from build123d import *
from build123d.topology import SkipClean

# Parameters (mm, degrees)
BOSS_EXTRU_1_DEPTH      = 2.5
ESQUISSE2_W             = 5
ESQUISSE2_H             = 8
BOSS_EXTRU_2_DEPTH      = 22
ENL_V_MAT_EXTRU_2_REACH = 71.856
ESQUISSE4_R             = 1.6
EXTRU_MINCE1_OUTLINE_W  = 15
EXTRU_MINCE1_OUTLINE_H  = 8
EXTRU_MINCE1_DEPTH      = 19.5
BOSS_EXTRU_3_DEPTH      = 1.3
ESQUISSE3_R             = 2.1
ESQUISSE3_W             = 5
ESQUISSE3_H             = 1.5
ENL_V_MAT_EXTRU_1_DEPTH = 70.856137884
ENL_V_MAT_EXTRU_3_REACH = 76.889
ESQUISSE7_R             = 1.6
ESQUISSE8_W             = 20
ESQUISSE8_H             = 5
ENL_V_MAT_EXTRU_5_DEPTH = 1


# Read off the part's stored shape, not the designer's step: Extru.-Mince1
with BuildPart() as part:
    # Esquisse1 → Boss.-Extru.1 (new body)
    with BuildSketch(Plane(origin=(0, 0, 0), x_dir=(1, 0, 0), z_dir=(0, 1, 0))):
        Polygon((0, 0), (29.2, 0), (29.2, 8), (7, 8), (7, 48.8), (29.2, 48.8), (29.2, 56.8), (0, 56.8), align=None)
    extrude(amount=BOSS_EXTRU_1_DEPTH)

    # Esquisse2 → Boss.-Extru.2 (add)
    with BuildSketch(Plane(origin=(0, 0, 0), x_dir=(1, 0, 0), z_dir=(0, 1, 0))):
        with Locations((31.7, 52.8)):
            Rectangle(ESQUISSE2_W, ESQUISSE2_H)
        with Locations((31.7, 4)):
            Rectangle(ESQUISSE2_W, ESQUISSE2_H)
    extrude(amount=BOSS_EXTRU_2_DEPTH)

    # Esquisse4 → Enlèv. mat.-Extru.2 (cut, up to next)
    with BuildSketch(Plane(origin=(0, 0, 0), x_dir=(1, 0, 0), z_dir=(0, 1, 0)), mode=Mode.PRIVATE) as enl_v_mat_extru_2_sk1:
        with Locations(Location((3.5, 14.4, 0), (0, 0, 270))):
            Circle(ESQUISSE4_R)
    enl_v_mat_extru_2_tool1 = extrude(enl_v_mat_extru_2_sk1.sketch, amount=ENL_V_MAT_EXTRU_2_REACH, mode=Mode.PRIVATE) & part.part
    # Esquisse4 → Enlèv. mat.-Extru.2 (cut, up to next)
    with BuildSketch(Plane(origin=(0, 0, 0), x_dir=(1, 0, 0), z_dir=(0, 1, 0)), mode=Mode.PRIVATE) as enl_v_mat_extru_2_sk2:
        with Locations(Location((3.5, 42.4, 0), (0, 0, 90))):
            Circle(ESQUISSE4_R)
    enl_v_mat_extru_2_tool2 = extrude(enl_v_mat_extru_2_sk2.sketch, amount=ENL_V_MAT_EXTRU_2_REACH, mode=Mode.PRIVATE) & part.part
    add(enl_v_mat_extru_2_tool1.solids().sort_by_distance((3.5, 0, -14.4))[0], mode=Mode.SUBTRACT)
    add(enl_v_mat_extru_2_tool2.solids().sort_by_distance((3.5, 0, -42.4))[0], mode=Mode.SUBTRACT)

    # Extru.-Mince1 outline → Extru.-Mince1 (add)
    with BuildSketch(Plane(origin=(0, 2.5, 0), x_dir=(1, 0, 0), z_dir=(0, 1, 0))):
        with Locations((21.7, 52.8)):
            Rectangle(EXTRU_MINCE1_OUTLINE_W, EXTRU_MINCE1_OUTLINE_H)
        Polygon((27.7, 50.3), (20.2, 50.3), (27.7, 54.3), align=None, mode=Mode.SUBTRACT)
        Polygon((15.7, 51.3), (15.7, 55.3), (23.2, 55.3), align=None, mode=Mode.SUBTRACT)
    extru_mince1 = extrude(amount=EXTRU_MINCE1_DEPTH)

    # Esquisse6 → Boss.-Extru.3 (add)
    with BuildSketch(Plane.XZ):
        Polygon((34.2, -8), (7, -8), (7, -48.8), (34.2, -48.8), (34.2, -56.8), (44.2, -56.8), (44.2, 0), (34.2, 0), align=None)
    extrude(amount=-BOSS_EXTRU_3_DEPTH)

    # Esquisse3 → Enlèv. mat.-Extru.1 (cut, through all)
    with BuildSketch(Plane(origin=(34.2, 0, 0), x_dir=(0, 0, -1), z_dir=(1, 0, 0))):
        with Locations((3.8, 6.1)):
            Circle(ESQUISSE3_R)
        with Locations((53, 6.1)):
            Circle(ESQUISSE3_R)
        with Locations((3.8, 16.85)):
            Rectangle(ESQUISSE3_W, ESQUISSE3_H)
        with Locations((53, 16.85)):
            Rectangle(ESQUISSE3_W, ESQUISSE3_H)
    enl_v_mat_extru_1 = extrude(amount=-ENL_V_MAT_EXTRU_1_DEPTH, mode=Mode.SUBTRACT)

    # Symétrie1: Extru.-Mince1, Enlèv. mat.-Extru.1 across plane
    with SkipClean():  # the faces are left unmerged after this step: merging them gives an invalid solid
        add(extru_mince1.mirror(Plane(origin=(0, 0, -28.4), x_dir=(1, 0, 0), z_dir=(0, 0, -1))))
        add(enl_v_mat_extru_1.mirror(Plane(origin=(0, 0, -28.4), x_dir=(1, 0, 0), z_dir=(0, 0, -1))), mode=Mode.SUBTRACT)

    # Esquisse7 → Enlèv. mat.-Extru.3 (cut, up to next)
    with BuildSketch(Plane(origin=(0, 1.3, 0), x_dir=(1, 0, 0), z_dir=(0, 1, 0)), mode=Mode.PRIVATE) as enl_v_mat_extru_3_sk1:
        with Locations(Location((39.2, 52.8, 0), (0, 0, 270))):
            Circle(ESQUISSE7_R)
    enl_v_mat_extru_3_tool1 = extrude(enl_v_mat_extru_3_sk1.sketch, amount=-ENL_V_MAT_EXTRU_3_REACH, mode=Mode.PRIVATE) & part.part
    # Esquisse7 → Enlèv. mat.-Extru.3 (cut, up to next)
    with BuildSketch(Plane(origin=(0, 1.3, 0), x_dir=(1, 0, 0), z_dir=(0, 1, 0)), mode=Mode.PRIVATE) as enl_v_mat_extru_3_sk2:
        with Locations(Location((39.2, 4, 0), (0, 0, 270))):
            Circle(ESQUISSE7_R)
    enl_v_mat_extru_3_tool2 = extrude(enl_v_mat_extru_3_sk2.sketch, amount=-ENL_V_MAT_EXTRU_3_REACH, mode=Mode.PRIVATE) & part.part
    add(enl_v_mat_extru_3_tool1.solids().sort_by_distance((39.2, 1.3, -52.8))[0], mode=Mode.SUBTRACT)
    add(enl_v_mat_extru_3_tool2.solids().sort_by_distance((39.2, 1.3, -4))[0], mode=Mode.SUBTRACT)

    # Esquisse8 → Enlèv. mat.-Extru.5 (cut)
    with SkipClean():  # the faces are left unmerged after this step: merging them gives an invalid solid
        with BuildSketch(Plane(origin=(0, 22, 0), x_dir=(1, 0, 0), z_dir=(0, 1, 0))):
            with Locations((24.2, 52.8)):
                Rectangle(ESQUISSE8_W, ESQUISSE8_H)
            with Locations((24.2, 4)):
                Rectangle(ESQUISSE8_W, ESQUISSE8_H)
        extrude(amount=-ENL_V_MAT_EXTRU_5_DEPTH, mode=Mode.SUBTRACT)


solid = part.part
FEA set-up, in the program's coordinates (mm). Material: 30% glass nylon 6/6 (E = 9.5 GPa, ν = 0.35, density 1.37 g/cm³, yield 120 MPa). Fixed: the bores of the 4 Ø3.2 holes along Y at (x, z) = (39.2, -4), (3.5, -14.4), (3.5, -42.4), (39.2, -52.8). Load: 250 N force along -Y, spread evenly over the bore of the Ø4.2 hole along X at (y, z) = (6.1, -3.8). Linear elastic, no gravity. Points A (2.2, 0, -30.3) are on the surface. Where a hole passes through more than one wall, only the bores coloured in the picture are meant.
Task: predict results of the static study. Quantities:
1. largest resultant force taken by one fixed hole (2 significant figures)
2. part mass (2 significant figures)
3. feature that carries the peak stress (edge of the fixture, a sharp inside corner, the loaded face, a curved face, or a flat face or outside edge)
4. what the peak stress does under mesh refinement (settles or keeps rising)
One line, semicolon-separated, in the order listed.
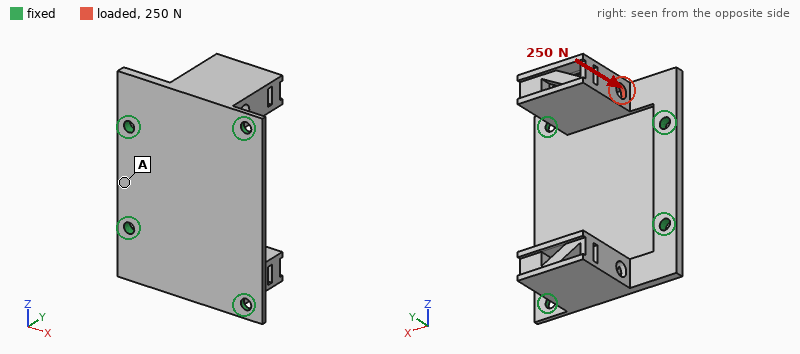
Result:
140 N; 12 g; edge of the fixture; keeps rising
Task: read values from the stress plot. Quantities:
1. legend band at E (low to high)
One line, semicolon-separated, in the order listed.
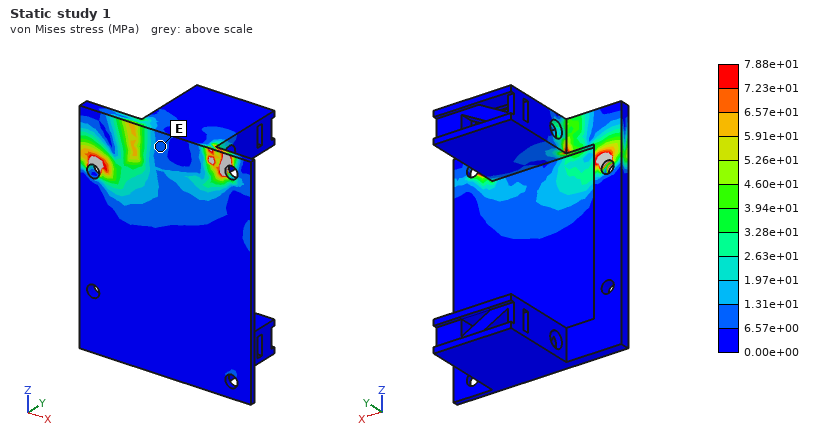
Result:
6.57e+00 to 1.31e+01 MPa
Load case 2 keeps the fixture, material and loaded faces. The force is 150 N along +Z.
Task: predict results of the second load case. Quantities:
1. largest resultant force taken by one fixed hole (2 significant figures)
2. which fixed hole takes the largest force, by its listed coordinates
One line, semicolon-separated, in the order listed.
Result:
63 N; (3.5, -14.4)
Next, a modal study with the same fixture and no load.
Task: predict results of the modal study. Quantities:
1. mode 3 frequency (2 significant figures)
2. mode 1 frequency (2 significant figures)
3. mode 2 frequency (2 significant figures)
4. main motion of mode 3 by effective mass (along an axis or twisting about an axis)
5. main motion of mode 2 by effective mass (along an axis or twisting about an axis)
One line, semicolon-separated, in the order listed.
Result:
2000 Hz; 1000 Hz; 1100 Hz; along Y; along Z
